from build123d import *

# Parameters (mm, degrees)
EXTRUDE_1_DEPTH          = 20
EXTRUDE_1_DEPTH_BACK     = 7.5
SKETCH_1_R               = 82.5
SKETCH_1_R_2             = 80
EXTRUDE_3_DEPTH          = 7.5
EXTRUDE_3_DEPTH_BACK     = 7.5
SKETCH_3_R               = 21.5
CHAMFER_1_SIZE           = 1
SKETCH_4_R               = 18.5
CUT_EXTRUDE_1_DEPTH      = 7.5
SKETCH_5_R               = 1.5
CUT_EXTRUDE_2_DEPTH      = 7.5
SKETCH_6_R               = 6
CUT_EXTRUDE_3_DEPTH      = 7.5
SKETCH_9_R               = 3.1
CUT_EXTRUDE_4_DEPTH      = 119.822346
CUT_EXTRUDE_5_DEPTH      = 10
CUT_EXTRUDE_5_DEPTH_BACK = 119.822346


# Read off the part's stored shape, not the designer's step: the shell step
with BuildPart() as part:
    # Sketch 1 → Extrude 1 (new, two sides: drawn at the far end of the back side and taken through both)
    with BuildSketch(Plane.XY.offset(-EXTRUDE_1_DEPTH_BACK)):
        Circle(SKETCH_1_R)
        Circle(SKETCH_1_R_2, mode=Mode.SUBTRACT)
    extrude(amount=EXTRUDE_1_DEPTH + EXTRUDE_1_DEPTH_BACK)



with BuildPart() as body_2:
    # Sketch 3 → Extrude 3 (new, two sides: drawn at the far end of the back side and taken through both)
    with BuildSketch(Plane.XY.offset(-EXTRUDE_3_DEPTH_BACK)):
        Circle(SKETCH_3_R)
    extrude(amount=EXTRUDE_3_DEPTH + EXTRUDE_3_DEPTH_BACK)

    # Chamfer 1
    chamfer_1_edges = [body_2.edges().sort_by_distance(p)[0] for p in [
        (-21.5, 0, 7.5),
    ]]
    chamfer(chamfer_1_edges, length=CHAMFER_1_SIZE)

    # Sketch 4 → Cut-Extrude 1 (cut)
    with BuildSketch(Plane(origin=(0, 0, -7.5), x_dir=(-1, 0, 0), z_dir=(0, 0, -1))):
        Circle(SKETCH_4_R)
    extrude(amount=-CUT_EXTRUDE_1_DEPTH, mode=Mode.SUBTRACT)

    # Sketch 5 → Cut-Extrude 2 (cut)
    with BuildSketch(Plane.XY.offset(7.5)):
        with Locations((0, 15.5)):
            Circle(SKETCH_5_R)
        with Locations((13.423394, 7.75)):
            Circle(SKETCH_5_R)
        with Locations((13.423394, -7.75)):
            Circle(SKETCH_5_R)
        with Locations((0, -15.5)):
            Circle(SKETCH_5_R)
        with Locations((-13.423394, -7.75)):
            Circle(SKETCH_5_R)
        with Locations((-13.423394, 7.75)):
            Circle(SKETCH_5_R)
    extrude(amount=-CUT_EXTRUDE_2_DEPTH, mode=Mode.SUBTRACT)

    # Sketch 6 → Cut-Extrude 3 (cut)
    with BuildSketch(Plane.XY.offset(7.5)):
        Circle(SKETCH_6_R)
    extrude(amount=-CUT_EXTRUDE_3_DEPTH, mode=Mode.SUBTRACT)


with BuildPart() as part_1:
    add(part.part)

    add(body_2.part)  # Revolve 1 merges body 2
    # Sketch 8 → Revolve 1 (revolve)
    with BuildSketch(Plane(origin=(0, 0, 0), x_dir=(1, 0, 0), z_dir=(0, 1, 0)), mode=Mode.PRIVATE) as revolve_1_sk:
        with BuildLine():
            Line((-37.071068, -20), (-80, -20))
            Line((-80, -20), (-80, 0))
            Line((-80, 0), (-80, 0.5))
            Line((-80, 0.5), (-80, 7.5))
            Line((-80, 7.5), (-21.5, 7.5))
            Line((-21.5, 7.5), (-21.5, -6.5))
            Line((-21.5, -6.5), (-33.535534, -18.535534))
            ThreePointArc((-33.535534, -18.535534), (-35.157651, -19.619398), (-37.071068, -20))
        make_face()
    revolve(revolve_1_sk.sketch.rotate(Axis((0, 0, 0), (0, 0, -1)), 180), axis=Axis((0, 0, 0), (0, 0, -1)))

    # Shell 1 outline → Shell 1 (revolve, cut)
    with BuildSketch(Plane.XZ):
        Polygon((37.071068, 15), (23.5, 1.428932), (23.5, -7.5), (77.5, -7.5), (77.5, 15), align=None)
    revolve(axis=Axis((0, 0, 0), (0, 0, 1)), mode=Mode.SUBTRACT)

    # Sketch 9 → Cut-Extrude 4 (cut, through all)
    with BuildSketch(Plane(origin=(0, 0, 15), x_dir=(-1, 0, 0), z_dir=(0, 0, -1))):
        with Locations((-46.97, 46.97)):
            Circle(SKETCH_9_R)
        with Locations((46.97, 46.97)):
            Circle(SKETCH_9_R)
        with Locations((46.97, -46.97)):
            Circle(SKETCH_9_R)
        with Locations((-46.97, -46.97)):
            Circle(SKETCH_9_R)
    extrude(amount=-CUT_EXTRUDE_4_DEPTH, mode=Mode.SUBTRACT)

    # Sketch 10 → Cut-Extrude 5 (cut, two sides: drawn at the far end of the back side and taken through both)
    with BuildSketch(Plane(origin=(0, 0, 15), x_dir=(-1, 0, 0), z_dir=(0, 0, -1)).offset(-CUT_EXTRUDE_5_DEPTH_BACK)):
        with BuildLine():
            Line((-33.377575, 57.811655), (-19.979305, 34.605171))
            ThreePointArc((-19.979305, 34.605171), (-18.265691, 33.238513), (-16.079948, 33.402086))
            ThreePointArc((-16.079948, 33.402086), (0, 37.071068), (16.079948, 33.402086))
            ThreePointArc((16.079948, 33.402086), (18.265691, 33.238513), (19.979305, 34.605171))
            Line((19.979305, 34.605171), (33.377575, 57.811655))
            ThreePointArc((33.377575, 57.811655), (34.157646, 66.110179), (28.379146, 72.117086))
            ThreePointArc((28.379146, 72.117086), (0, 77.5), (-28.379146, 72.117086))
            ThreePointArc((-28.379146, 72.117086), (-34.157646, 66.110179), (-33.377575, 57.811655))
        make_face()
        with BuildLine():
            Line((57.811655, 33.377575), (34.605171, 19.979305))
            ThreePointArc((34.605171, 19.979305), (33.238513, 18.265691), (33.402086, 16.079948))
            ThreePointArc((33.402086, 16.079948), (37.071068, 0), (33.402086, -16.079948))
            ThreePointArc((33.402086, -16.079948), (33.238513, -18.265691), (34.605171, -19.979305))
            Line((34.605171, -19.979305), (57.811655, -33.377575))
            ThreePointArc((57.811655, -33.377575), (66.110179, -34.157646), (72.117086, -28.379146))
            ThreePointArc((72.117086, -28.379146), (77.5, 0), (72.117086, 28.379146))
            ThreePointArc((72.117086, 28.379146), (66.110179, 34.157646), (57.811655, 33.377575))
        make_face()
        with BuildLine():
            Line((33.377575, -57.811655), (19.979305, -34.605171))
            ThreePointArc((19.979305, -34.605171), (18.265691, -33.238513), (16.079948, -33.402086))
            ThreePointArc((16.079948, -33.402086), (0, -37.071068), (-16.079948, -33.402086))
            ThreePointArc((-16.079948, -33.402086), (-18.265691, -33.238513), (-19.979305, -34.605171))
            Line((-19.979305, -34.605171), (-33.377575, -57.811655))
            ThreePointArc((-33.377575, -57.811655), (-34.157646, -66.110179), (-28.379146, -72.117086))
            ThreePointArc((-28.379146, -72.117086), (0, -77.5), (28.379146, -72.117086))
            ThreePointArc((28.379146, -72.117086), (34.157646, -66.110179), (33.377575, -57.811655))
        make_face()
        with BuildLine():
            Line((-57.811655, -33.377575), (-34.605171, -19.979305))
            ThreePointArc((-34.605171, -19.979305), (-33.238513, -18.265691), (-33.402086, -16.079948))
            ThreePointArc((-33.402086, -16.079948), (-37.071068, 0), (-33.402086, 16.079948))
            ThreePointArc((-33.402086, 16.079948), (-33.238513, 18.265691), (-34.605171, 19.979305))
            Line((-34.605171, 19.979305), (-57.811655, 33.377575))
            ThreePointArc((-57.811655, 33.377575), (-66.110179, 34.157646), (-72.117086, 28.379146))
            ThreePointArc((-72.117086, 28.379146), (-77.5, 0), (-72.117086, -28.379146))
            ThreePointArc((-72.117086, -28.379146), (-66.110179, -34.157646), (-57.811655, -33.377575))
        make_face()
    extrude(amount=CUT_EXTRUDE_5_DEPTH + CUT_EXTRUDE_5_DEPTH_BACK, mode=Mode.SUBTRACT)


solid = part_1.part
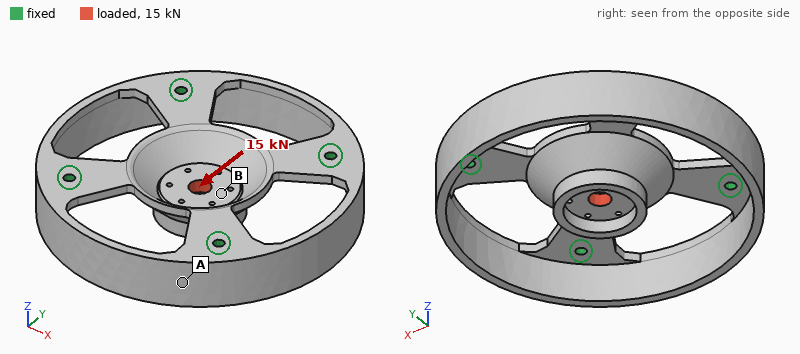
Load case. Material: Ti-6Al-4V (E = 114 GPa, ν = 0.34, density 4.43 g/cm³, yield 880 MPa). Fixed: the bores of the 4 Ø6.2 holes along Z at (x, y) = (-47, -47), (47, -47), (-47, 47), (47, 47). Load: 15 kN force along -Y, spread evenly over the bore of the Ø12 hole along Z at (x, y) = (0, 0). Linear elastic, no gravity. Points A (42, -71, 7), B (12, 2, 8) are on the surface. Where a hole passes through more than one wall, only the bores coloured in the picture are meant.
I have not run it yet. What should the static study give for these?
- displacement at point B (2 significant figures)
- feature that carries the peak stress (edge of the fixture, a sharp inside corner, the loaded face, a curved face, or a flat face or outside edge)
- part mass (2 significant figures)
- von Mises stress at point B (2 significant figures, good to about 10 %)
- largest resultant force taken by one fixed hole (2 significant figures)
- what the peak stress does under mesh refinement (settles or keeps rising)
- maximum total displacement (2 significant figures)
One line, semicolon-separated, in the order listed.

0.072 mm; edge of the fixture; 570 g; 48 MPa; 4.7 kN; keeps rising; 0.14 mm
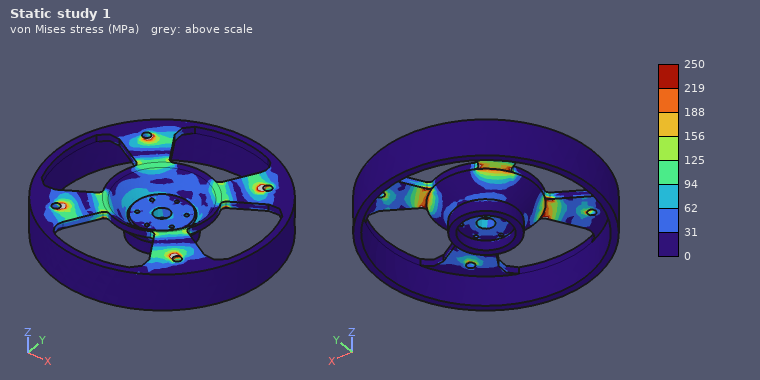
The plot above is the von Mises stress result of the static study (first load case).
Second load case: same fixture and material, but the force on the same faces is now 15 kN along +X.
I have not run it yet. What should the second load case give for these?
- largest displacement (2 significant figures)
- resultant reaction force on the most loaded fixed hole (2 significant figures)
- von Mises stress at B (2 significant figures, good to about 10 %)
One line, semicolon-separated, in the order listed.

0.14 mm; 4.7 kN; 39 MPa
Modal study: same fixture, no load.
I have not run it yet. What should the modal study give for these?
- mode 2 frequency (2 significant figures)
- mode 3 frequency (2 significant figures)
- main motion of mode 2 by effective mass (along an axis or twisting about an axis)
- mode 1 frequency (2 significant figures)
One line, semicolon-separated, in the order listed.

2300 Hz; 2900 Hz; along Z; 1600 Hz
